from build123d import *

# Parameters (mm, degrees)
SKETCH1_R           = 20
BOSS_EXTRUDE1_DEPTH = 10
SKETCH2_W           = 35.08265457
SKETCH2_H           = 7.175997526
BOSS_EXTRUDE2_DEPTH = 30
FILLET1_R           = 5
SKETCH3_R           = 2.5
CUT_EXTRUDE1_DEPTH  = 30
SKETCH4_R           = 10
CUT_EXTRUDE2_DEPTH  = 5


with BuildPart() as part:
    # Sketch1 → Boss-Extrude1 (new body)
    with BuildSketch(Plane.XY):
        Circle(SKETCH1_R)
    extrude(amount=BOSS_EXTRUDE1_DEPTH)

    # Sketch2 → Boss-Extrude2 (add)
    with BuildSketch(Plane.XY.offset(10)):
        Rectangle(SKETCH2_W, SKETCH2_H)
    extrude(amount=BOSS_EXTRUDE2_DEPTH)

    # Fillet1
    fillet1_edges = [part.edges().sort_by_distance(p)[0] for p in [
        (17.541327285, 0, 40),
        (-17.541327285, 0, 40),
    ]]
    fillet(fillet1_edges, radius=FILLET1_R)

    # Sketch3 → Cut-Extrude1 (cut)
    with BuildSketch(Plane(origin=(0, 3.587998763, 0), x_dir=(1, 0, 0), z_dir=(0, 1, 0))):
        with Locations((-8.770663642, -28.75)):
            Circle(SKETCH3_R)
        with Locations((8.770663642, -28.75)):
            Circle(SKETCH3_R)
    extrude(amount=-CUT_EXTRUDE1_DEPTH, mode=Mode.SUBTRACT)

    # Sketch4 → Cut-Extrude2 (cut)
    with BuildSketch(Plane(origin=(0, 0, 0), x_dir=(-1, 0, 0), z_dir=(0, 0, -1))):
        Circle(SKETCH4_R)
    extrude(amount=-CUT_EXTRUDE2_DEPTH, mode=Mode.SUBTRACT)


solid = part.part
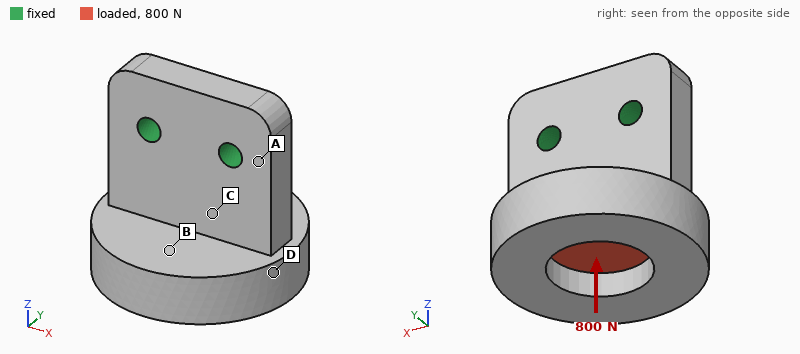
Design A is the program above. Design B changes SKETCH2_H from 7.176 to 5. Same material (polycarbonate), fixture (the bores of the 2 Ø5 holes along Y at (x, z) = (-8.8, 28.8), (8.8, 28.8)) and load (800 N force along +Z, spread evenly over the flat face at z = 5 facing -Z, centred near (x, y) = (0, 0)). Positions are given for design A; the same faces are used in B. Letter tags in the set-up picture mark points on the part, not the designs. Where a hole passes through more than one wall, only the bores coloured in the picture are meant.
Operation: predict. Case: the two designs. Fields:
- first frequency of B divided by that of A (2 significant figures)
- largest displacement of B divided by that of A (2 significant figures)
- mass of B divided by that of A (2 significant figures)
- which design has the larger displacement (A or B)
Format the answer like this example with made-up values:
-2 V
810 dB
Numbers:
0.61
1.4
0.88
B
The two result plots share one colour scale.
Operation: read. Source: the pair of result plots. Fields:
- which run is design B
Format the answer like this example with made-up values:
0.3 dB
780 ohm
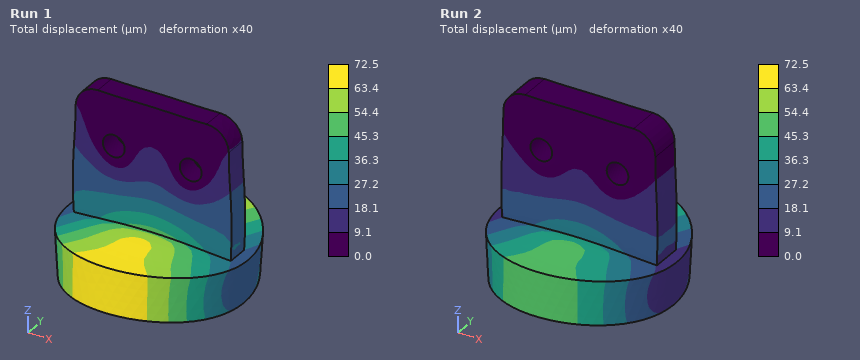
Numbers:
Run 1
